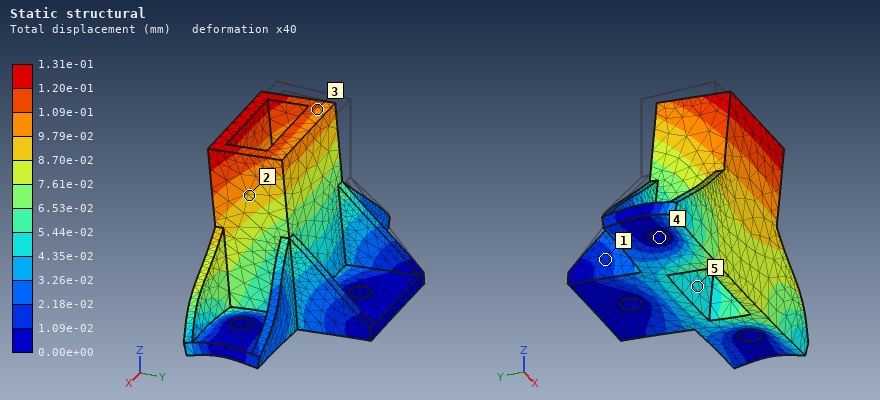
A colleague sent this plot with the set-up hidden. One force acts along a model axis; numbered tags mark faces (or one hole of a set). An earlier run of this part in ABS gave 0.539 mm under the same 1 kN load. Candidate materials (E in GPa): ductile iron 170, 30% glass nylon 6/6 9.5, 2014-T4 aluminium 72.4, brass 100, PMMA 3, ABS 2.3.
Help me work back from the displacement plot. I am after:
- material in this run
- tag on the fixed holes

30% glass nylon 6/6
4
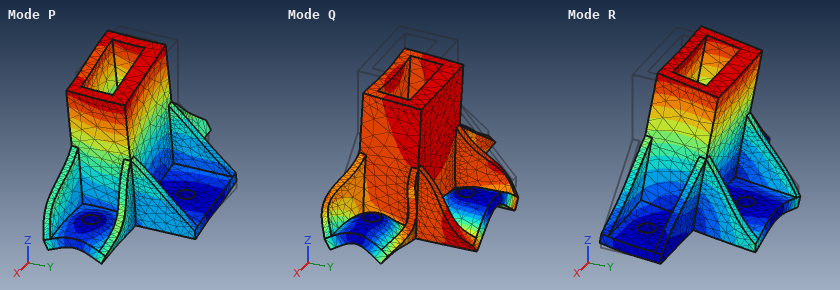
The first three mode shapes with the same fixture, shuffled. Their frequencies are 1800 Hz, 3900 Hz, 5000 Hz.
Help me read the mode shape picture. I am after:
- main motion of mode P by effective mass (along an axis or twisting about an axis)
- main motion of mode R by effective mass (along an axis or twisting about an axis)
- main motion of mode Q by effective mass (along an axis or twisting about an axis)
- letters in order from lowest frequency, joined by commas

along X
along Y
along Z
R, P, Q
